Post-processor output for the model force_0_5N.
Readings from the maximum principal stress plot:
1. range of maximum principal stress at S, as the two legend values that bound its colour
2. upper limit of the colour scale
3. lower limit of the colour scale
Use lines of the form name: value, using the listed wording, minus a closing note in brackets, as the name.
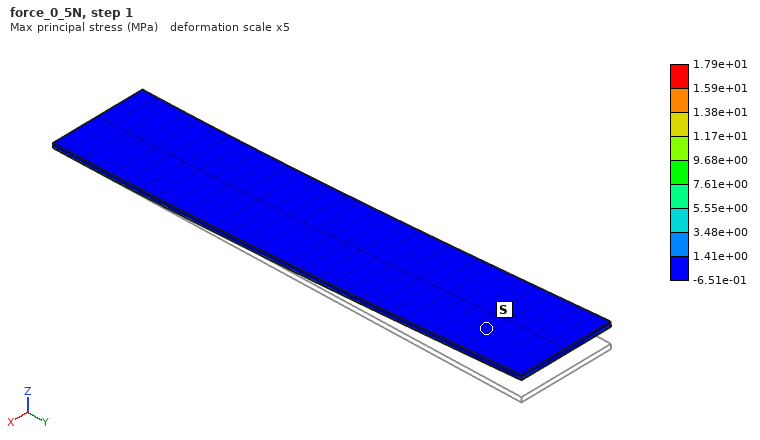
range of maximum principal stress at S, as the two legend values that bound its colour: -6.51e-01 to 1.41e+00 MPa
upper limit of the colour scale: 1.79e+01 MPa
lower limit of the colour scale: -6.51e-01 MPa
